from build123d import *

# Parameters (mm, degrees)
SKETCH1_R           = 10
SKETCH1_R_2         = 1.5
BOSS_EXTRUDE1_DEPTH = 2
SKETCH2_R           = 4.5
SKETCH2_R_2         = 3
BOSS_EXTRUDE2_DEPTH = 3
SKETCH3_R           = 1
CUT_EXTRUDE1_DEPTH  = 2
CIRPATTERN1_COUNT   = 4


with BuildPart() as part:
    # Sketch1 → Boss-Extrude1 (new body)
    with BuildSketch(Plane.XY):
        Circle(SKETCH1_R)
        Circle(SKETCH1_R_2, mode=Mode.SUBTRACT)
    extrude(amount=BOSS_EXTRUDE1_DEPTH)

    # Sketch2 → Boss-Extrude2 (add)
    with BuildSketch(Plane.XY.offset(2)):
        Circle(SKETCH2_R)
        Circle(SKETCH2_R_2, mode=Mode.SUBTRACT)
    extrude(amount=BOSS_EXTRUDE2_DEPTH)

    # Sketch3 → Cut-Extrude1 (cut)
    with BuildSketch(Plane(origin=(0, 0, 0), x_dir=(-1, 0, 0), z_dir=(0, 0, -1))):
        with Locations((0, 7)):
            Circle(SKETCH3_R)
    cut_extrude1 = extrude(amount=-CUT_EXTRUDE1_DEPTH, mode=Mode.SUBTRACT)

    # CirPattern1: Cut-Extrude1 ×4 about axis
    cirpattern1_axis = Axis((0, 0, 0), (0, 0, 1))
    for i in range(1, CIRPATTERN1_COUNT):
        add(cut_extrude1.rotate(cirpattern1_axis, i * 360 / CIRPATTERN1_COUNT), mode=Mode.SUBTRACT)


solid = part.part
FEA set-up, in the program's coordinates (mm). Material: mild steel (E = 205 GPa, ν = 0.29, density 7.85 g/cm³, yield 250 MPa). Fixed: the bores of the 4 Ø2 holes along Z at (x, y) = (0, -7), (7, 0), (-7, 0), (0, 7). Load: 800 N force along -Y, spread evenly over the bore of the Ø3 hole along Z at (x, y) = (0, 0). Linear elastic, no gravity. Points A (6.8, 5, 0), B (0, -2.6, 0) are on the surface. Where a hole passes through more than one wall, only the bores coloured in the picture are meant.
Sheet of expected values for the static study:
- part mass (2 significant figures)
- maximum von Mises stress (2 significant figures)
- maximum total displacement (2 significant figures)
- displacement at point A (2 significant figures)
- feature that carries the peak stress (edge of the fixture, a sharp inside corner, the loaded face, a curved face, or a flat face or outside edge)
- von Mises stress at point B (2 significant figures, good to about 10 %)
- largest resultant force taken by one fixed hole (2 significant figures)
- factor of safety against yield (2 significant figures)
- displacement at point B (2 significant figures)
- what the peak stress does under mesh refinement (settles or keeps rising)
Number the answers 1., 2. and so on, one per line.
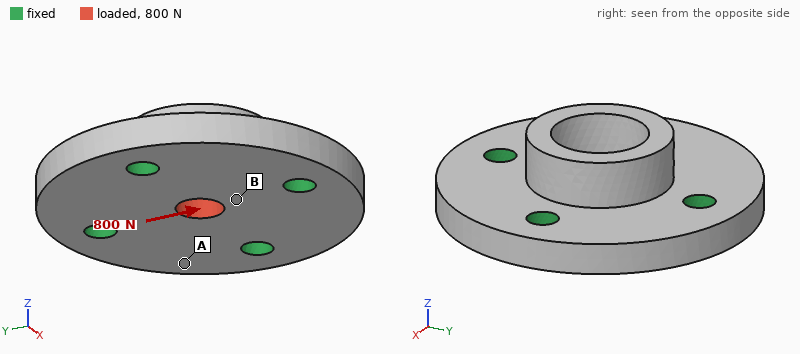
1. 5.5 g
2. 75 MPa
3. 0.91 µm
4. 0.21 µm
5. the loaded face
6. 43 MPa
7. 270 N
8. 3.3
9. 0.65 µm
10. settles
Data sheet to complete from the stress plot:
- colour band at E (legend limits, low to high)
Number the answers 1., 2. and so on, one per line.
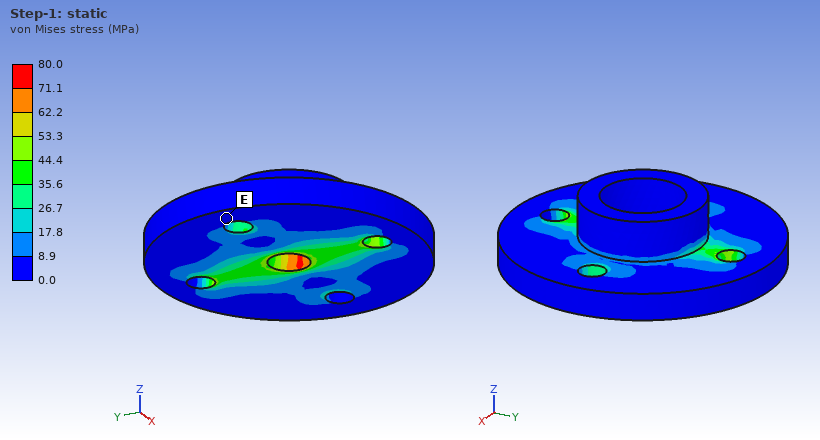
1. 0.0 to 8.9 MPa
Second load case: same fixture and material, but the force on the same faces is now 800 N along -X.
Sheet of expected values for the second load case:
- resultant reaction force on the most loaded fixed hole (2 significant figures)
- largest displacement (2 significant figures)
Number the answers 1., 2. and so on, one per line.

1. 270 N
2. 0.91 µm
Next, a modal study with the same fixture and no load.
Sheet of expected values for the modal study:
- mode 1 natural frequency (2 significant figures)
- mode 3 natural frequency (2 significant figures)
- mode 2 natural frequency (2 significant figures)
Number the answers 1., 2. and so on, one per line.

1. 63 kHz
2. 65 kHz
3. 65 kHz
